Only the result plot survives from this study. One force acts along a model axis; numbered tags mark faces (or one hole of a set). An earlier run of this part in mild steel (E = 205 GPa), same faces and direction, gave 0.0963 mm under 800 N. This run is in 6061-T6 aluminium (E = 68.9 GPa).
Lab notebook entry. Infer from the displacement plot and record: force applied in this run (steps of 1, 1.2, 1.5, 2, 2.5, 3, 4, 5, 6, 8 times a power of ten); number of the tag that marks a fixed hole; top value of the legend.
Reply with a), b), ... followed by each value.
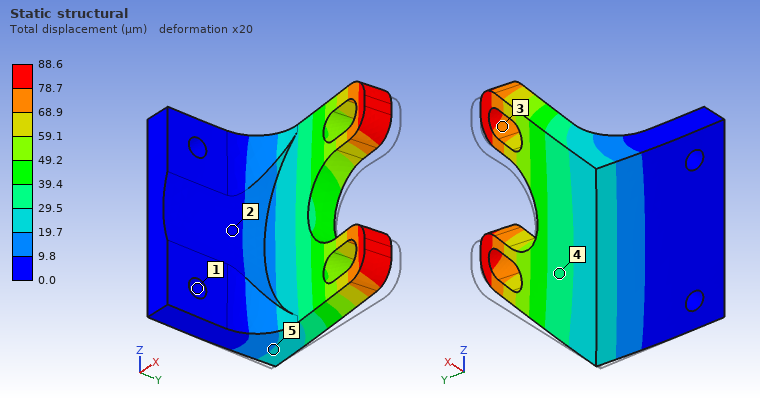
a) 250 N
b) 1
c) 88.6 µm
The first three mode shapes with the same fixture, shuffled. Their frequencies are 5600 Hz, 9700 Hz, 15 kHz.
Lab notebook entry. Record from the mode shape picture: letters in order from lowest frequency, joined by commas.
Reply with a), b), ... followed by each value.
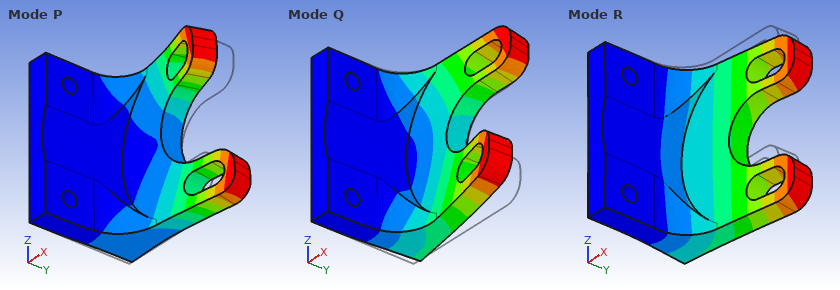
a) R, Q, P
